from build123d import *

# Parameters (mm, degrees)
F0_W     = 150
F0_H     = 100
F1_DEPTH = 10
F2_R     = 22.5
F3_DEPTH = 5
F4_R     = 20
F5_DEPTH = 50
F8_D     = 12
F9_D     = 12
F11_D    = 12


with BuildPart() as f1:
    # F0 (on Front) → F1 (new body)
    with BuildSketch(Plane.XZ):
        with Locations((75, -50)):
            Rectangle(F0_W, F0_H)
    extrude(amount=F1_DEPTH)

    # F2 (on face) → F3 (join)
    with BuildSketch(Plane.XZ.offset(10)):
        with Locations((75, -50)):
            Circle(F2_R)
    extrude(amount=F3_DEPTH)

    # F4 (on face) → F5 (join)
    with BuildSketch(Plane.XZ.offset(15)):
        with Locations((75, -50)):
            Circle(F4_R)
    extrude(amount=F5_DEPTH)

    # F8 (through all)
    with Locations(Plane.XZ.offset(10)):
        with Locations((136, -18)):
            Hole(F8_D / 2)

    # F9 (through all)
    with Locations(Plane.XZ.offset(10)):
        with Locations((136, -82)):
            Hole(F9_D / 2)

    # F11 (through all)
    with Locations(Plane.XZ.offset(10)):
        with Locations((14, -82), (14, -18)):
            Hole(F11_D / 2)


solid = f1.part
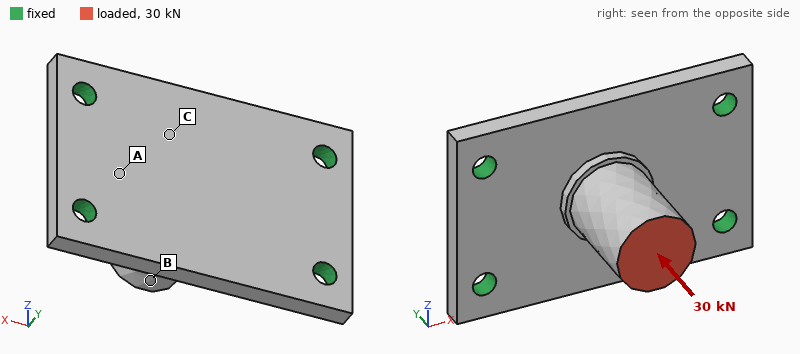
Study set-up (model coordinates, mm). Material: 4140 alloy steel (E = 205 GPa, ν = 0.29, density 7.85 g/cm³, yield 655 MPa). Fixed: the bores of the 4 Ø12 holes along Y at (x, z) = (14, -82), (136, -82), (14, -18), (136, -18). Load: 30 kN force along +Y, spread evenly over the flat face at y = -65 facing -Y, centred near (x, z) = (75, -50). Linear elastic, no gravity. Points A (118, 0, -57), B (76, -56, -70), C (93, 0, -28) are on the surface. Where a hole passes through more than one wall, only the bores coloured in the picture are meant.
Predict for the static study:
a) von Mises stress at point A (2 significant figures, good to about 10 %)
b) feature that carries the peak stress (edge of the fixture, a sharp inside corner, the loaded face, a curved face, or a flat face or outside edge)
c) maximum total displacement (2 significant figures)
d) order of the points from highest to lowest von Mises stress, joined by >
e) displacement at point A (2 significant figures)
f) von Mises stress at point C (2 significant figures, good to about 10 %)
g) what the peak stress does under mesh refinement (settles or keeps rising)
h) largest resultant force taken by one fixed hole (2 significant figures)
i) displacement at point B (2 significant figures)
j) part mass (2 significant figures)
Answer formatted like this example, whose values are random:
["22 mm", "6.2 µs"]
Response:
["75 MPa", "edge of the fixture", "0.12 mm", "C > A > B", "0.050 mm", "120 MPa", "keeps rising", "7.9 kN", "0.12 mm", "1.7 kg"]
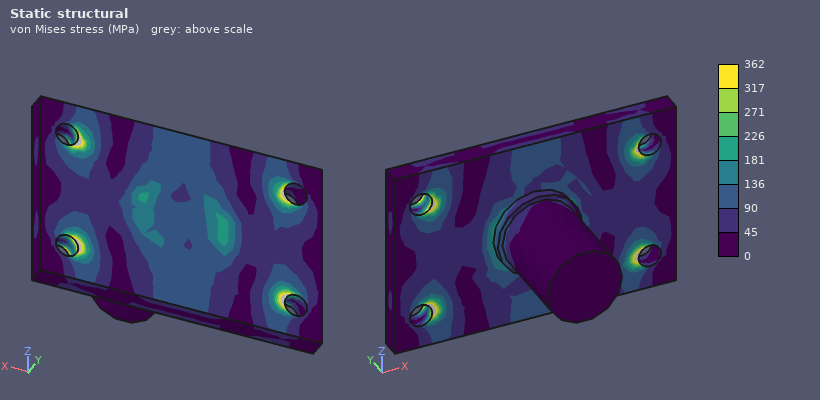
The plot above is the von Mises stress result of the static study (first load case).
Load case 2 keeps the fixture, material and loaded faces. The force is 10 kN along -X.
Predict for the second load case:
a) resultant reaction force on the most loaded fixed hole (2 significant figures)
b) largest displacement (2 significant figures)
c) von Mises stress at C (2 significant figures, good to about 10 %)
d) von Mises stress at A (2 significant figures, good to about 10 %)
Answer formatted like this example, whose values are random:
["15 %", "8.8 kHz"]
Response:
["4.3 kN", "0.12 mm", "75 MPa", "34 MPa"]
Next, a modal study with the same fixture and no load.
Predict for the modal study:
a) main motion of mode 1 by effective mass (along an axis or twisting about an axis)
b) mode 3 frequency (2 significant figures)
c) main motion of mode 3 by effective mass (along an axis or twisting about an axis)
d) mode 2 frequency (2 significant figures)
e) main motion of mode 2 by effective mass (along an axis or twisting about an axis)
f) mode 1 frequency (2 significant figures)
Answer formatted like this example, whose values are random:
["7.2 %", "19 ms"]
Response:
["along Z", "3200 Hz", "along X", "2600 Hz", "along Y", "2400 Hz"]
